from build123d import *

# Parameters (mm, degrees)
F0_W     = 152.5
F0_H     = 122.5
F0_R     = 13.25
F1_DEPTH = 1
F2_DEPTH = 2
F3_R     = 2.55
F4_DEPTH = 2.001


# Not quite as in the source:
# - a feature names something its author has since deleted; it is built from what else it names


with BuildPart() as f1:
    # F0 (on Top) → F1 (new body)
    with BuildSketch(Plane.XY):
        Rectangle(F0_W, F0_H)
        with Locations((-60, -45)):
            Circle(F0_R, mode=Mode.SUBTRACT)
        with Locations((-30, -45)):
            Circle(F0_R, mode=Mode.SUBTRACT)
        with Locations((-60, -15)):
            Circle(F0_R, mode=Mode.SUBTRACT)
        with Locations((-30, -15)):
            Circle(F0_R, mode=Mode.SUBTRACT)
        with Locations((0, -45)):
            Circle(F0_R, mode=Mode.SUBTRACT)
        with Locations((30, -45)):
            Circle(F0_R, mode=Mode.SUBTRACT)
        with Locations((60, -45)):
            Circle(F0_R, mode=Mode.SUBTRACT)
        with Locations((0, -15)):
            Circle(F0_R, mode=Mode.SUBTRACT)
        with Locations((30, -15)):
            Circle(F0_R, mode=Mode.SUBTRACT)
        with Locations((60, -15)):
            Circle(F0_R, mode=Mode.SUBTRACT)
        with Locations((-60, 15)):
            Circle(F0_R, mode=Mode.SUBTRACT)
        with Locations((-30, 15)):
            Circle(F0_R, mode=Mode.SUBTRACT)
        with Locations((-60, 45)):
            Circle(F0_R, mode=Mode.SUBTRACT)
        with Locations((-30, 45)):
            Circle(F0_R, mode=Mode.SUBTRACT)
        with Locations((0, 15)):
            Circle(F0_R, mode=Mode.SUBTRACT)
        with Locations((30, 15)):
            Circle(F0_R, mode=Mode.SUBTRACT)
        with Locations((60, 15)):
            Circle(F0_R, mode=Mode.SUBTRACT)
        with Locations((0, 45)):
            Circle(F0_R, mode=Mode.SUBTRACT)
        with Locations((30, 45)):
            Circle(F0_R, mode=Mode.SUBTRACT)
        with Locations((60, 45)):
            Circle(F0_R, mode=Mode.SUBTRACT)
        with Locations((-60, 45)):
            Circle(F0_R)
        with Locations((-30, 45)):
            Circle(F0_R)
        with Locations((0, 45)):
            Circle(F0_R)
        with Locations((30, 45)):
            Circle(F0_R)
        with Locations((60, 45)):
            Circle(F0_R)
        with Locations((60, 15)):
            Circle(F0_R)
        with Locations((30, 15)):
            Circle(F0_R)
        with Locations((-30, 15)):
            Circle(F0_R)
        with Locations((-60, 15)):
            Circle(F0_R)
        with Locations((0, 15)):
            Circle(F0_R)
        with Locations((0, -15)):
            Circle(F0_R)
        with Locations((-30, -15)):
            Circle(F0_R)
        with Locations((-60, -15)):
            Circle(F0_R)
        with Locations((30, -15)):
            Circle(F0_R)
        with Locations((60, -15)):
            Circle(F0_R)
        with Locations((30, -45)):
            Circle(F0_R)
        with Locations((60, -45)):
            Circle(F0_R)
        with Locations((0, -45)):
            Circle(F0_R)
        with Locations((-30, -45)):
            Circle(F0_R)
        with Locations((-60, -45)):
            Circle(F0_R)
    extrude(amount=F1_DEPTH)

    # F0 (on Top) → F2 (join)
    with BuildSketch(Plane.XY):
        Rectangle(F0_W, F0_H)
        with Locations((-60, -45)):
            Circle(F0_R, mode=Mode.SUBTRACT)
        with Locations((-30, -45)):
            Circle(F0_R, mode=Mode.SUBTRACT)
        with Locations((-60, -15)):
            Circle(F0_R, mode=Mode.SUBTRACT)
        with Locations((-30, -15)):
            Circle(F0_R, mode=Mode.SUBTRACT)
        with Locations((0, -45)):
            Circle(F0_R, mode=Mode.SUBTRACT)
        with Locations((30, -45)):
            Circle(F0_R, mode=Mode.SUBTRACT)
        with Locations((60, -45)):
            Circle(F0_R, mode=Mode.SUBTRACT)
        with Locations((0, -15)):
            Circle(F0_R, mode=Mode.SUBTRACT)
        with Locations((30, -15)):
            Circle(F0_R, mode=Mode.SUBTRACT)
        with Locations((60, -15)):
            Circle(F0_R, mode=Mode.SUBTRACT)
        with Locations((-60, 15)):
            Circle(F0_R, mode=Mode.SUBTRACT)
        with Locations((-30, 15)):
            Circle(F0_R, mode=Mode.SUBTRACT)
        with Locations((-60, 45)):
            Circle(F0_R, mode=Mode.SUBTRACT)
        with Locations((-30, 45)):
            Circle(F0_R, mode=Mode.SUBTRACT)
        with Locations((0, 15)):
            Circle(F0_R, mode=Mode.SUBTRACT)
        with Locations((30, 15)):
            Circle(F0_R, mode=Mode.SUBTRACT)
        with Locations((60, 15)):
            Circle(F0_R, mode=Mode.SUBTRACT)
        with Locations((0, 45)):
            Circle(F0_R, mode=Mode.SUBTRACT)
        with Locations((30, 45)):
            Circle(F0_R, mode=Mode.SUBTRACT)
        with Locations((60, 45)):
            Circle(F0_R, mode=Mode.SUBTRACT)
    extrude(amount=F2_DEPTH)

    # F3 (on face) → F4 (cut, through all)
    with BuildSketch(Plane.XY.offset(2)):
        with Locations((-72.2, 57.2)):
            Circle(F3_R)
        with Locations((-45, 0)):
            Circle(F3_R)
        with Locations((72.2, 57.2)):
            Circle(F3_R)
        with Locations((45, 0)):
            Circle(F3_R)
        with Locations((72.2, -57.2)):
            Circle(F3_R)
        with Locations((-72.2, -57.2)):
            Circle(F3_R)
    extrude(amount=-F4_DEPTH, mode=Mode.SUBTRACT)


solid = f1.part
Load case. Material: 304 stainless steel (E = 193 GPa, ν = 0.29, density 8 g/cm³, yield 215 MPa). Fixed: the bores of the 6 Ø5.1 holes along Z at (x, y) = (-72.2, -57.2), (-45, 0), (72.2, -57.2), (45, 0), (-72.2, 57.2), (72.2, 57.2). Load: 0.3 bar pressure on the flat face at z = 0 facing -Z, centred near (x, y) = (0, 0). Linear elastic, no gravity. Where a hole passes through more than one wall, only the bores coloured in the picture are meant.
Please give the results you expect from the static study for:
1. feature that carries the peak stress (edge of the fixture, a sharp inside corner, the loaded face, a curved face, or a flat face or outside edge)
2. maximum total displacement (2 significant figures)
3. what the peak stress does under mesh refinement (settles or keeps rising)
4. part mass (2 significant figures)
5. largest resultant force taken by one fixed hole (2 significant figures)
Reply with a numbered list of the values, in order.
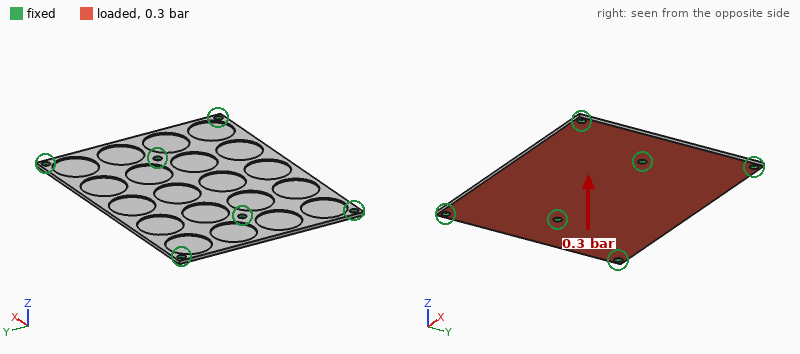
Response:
1. edge of the fixture
2. 0.36 mm
3. keeps rising
4. 210 g
5. 180 N
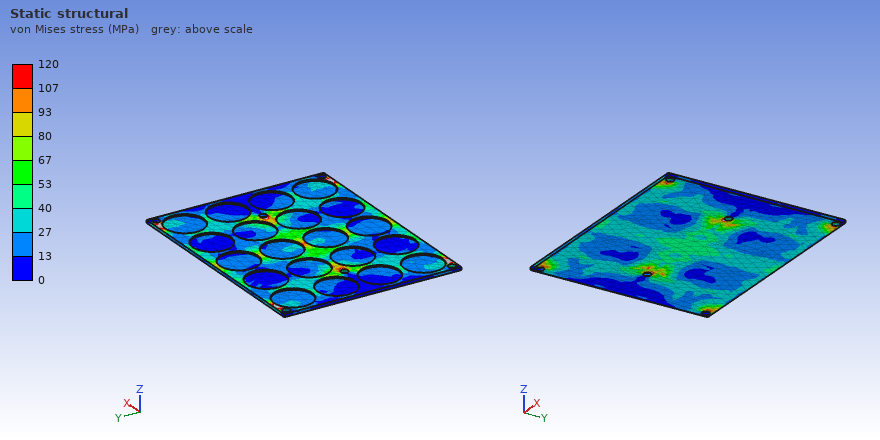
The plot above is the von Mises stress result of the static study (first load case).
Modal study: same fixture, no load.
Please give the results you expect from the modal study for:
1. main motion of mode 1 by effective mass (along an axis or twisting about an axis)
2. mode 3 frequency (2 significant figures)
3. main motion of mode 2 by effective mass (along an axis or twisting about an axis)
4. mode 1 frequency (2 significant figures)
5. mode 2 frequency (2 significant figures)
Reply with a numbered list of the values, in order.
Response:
1. twisting about X
2. 1200 Hz
3. along Z
4. 530 Hz
5. 560 Hz
